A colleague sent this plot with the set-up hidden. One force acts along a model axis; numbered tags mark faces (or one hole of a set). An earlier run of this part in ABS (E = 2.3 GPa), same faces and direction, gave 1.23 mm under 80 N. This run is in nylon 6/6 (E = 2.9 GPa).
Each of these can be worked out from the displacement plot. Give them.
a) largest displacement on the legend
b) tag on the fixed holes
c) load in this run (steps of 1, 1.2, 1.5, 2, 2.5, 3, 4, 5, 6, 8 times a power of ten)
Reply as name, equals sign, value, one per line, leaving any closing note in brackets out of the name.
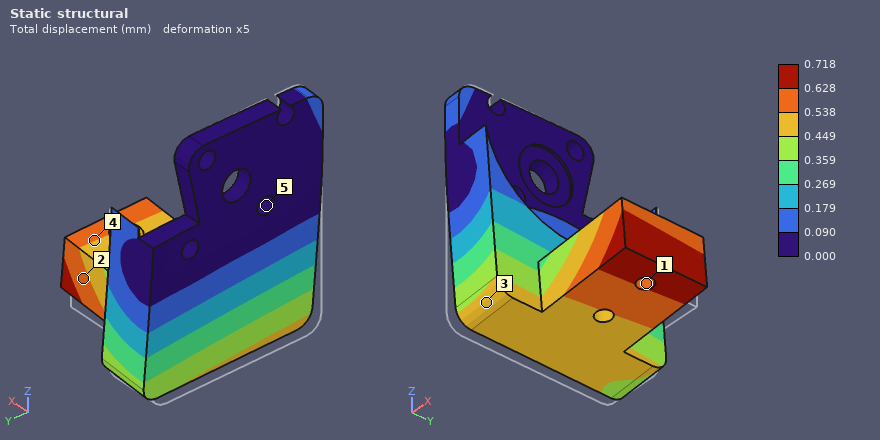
largest displacement on the legend = 0.718 mm
tag on the fixed holes = 5
load in this run = 60 N
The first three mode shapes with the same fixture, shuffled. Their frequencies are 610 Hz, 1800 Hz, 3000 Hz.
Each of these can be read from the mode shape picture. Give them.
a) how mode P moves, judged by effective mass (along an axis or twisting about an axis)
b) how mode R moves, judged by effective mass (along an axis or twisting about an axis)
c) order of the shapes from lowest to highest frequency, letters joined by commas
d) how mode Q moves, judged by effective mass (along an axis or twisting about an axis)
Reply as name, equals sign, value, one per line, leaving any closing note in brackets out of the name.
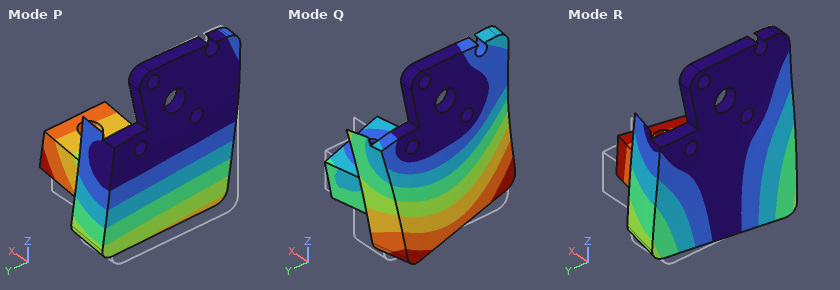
how mode P moves, judged by effective mass = along X
how mode R moves, judged by effective mass = along Y
order of the shapes from lowest to highest frequency, letters joined by commas = P, R, Q
how mode Q moves, judged by effective mass = along Y
